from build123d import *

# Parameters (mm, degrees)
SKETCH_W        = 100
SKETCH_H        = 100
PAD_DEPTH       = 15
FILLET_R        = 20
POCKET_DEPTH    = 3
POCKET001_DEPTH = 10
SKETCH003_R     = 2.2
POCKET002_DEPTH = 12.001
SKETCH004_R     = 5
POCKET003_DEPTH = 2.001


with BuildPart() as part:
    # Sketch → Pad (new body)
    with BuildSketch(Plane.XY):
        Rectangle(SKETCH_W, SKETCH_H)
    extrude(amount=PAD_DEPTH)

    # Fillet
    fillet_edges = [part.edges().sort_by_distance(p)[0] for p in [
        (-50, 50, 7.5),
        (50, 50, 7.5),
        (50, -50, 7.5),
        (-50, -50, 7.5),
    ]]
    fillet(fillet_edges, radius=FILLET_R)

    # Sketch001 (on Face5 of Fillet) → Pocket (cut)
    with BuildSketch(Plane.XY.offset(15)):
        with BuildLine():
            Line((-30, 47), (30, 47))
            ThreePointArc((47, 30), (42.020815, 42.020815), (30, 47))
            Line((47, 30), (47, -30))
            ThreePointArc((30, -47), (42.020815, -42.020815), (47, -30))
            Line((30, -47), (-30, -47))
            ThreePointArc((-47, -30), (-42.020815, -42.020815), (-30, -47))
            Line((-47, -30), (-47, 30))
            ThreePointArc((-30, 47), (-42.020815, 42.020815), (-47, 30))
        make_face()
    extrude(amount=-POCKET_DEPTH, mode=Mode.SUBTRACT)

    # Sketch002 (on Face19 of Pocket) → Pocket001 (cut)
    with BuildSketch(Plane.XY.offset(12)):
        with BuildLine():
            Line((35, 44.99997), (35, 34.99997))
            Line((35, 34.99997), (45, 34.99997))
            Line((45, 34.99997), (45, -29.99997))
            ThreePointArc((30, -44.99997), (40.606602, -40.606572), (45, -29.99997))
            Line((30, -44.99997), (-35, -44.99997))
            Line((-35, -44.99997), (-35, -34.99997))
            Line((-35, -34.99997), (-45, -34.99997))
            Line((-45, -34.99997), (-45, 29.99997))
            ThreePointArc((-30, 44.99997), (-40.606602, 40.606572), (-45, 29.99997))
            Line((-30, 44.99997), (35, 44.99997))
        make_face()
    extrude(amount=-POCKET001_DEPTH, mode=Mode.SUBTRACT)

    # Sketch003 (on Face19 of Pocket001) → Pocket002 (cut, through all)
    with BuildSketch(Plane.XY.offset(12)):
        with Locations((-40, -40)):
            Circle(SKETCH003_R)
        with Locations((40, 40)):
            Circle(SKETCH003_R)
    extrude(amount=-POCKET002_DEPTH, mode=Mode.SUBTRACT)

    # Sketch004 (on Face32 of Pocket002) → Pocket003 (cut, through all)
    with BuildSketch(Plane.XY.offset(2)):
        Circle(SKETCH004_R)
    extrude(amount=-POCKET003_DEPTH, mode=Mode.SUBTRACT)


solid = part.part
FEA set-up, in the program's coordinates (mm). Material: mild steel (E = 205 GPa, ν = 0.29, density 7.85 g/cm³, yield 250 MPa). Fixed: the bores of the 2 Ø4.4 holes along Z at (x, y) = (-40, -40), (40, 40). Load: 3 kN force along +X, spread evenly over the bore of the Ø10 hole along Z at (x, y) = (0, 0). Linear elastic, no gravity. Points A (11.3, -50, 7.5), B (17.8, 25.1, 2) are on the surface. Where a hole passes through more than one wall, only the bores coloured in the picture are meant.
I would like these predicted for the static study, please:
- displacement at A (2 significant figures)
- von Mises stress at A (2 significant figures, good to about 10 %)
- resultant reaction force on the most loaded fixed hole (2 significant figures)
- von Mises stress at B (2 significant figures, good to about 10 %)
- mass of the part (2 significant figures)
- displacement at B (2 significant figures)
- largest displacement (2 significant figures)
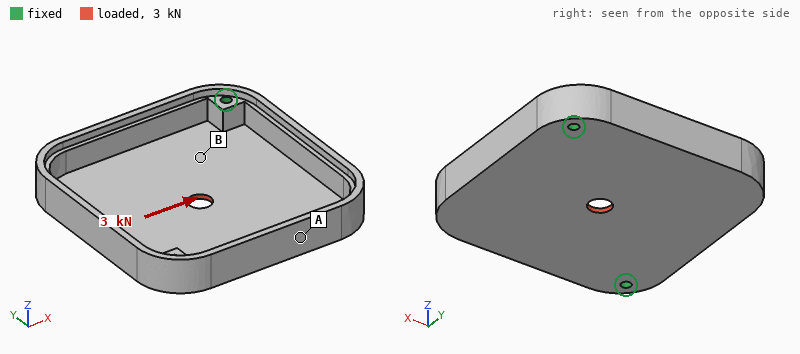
9.7 µm
5.7 MPa
1.5 kN
19 MPa
320 g
4.7 µm
19 µm
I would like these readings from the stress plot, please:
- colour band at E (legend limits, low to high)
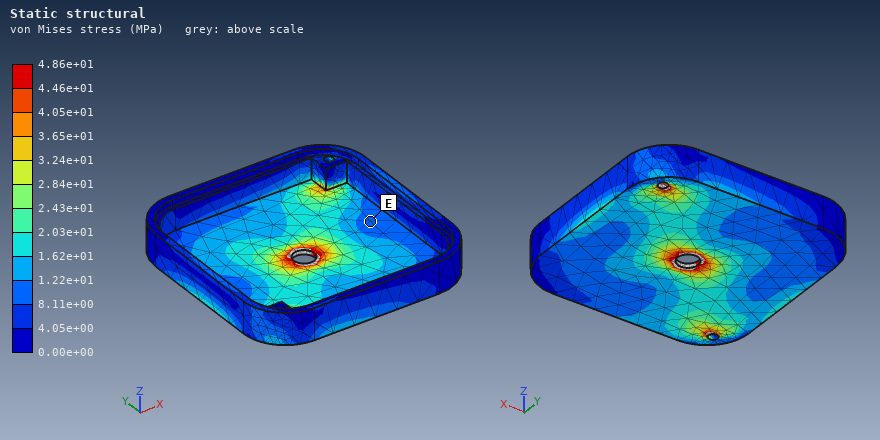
8.11e+00 to 1.22e+01 MPa
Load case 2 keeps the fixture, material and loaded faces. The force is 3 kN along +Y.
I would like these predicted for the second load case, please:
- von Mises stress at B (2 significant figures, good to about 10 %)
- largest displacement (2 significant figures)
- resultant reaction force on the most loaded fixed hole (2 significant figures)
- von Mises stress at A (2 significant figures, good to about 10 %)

18 MPa
19 µm
1.5 kN
5.6 MPa
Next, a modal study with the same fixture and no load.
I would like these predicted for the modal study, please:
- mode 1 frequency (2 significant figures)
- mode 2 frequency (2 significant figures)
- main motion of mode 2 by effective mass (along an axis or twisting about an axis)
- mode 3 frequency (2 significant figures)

1600 Hz
1600 Hz
along Z
2200 Hz
